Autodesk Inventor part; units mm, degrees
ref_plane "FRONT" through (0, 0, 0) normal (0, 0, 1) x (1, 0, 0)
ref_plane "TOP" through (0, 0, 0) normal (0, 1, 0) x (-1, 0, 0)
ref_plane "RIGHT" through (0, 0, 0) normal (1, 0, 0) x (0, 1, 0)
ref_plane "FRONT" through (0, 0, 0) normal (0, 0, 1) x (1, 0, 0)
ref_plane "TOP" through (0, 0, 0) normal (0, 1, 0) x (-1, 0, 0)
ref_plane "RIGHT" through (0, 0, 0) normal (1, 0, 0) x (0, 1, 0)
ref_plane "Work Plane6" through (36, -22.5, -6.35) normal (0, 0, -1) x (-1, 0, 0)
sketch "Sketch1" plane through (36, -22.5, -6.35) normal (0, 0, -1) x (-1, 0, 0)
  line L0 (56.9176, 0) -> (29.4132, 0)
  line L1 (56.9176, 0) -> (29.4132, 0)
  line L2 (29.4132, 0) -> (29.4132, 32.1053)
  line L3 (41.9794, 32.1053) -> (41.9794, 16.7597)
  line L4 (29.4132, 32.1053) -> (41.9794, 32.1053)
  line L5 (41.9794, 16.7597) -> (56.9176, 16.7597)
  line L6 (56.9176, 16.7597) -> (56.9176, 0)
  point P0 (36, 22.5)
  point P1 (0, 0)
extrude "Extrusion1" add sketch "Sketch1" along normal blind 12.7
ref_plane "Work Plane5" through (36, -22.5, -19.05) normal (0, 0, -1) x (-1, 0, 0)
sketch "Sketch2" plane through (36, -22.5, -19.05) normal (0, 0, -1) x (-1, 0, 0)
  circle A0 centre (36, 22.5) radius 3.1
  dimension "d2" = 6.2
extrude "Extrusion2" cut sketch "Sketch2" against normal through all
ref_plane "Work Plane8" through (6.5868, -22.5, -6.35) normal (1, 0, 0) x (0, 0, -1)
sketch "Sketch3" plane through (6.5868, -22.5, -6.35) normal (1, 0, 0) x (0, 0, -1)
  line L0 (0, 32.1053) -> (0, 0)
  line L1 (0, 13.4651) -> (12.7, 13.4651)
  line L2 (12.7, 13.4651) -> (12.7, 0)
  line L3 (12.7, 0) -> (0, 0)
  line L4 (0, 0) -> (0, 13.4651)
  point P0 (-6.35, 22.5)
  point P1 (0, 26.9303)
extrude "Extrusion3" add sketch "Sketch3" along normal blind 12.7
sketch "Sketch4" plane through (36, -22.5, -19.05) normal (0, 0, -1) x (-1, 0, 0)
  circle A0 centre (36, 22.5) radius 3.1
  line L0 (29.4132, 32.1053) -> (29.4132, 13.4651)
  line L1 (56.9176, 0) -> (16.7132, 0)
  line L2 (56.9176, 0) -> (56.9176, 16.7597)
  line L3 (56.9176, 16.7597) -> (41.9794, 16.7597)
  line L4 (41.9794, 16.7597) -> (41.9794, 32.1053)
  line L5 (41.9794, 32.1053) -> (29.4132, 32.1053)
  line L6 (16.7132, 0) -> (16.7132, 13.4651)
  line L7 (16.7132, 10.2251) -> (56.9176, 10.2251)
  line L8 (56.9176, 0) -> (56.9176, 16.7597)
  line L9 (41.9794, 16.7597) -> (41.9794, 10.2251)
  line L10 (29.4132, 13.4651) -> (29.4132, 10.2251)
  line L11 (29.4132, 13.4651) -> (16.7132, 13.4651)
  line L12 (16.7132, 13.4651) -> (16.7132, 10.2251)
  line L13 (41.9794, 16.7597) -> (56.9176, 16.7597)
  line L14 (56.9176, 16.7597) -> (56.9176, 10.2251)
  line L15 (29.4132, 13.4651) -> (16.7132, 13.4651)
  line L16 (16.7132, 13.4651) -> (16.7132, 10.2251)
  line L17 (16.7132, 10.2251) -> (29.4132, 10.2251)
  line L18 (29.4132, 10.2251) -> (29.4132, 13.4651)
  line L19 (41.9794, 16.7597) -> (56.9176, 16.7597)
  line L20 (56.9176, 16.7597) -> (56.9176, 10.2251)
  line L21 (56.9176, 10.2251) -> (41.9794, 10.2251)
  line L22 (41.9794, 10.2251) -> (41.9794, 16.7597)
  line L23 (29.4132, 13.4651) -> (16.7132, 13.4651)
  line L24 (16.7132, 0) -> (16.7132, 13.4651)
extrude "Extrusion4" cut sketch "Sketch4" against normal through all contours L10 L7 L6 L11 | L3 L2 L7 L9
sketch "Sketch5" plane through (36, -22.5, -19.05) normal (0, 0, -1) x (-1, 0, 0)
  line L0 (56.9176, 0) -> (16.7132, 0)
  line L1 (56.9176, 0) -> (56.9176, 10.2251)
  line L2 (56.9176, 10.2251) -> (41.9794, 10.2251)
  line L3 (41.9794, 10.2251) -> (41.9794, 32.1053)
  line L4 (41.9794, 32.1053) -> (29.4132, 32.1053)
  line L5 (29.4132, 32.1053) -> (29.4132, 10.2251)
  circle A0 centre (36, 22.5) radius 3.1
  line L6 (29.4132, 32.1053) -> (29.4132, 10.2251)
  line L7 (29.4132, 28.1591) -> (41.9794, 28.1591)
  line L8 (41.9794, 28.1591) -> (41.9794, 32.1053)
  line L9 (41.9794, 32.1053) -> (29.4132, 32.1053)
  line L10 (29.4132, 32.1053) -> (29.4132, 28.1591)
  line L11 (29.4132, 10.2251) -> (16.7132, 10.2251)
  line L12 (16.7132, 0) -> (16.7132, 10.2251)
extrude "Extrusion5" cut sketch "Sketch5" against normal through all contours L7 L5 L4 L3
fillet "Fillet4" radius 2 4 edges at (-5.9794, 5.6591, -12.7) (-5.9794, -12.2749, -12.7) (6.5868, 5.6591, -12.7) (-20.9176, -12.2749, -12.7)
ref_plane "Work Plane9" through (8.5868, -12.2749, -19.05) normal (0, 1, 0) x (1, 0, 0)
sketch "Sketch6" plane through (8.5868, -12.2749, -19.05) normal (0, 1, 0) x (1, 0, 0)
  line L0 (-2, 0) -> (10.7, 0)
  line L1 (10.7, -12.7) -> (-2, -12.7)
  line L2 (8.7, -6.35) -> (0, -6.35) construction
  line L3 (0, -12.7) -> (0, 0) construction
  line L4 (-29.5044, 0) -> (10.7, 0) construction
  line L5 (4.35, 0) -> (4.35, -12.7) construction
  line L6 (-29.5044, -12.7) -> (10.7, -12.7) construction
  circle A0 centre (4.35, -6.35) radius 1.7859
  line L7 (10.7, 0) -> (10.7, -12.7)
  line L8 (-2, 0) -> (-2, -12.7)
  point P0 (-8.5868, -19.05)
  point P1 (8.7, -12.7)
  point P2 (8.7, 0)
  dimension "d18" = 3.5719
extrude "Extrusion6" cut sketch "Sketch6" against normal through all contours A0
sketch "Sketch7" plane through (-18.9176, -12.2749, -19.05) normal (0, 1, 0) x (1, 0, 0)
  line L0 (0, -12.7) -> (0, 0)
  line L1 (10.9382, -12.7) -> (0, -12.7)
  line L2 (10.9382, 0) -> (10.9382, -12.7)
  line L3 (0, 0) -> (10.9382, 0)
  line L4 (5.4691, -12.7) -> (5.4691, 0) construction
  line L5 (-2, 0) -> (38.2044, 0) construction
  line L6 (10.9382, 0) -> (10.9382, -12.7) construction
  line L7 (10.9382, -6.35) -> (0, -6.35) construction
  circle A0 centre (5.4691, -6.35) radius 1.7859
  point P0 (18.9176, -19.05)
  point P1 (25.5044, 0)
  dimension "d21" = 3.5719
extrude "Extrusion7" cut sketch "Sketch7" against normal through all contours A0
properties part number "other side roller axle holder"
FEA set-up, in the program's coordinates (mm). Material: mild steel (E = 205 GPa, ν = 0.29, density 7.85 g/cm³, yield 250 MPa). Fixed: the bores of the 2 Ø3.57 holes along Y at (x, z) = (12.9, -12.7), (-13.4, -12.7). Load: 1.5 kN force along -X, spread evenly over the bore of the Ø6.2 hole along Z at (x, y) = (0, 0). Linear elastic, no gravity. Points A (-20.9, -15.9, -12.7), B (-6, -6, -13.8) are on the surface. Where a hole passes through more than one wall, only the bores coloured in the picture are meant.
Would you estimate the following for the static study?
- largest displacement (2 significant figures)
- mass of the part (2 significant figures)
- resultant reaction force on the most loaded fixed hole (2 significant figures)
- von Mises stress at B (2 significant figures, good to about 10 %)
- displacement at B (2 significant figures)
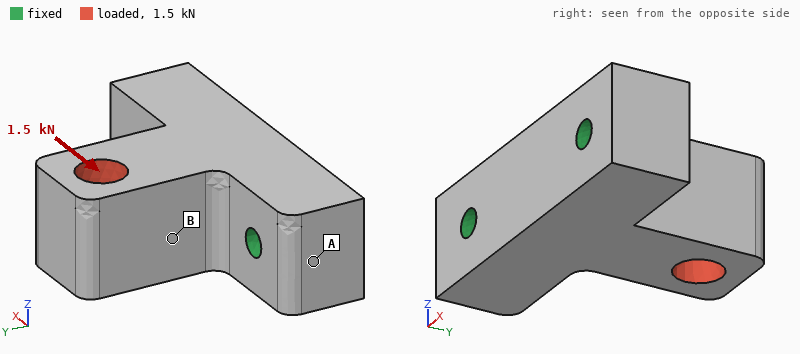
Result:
12 µm
59 g
1.4 kN
35 MPa
4.5 µm
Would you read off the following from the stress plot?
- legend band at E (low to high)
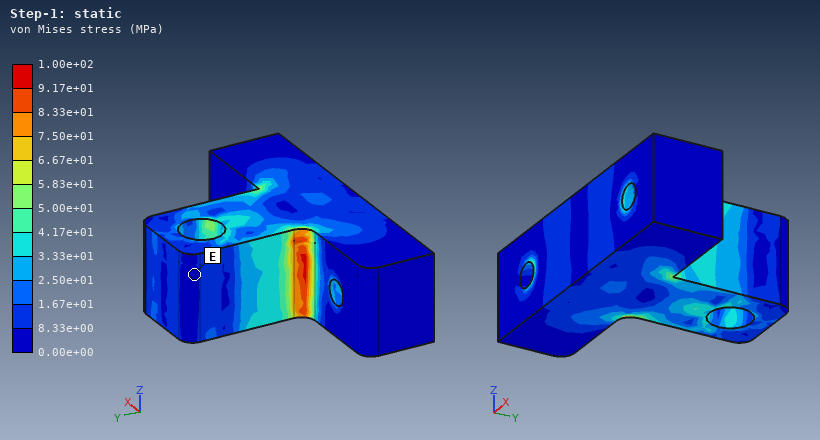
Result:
0.00e+00 to 8.33e+00 MPa
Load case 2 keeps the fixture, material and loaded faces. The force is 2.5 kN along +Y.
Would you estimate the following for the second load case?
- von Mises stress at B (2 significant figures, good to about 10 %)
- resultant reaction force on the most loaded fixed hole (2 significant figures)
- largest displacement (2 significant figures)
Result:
24 MPa
1.3 kN
3.9 µm
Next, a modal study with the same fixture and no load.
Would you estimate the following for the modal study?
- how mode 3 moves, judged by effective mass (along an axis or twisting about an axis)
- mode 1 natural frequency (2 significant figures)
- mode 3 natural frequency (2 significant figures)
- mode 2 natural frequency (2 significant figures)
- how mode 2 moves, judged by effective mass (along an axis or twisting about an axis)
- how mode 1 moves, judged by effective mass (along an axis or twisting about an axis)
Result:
along Y
12 kHz
31 kHz
19 kHz
along X
along Z
